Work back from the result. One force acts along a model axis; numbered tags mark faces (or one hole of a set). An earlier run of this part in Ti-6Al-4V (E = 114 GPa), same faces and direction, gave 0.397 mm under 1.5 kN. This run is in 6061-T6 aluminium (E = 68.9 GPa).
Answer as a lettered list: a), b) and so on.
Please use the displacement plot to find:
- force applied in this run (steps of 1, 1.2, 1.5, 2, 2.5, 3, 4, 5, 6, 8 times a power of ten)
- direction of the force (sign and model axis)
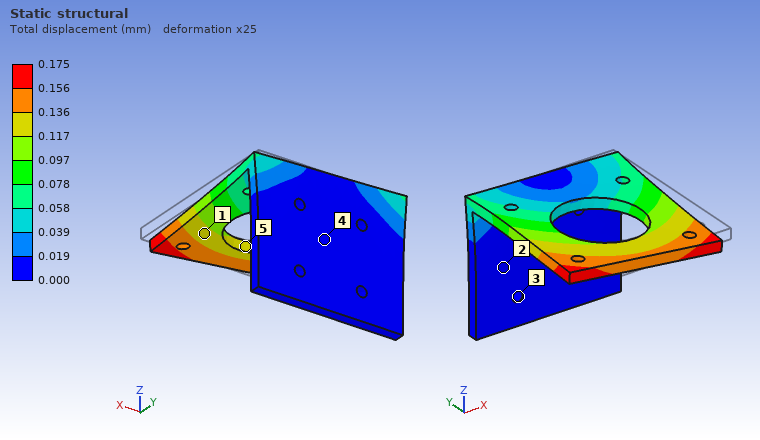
a) 400 N
b) -X
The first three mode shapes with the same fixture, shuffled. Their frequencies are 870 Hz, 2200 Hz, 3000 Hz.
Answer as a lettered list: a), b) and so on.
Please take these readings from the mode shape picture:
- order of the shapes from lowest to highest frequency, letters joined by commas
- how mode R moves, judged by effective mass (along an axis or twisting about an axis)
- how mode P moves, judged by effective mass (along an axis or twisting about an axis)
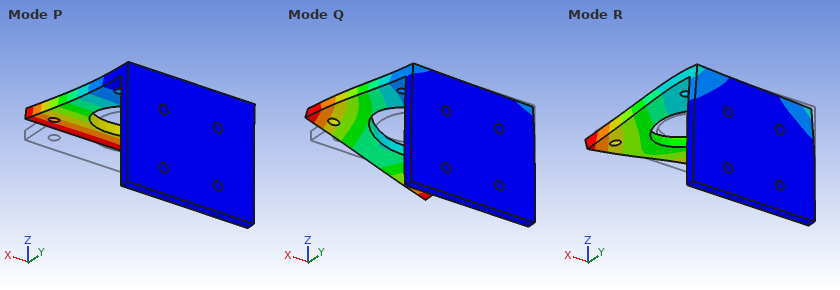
a) P, Q, R
b) along X
c) along Z
